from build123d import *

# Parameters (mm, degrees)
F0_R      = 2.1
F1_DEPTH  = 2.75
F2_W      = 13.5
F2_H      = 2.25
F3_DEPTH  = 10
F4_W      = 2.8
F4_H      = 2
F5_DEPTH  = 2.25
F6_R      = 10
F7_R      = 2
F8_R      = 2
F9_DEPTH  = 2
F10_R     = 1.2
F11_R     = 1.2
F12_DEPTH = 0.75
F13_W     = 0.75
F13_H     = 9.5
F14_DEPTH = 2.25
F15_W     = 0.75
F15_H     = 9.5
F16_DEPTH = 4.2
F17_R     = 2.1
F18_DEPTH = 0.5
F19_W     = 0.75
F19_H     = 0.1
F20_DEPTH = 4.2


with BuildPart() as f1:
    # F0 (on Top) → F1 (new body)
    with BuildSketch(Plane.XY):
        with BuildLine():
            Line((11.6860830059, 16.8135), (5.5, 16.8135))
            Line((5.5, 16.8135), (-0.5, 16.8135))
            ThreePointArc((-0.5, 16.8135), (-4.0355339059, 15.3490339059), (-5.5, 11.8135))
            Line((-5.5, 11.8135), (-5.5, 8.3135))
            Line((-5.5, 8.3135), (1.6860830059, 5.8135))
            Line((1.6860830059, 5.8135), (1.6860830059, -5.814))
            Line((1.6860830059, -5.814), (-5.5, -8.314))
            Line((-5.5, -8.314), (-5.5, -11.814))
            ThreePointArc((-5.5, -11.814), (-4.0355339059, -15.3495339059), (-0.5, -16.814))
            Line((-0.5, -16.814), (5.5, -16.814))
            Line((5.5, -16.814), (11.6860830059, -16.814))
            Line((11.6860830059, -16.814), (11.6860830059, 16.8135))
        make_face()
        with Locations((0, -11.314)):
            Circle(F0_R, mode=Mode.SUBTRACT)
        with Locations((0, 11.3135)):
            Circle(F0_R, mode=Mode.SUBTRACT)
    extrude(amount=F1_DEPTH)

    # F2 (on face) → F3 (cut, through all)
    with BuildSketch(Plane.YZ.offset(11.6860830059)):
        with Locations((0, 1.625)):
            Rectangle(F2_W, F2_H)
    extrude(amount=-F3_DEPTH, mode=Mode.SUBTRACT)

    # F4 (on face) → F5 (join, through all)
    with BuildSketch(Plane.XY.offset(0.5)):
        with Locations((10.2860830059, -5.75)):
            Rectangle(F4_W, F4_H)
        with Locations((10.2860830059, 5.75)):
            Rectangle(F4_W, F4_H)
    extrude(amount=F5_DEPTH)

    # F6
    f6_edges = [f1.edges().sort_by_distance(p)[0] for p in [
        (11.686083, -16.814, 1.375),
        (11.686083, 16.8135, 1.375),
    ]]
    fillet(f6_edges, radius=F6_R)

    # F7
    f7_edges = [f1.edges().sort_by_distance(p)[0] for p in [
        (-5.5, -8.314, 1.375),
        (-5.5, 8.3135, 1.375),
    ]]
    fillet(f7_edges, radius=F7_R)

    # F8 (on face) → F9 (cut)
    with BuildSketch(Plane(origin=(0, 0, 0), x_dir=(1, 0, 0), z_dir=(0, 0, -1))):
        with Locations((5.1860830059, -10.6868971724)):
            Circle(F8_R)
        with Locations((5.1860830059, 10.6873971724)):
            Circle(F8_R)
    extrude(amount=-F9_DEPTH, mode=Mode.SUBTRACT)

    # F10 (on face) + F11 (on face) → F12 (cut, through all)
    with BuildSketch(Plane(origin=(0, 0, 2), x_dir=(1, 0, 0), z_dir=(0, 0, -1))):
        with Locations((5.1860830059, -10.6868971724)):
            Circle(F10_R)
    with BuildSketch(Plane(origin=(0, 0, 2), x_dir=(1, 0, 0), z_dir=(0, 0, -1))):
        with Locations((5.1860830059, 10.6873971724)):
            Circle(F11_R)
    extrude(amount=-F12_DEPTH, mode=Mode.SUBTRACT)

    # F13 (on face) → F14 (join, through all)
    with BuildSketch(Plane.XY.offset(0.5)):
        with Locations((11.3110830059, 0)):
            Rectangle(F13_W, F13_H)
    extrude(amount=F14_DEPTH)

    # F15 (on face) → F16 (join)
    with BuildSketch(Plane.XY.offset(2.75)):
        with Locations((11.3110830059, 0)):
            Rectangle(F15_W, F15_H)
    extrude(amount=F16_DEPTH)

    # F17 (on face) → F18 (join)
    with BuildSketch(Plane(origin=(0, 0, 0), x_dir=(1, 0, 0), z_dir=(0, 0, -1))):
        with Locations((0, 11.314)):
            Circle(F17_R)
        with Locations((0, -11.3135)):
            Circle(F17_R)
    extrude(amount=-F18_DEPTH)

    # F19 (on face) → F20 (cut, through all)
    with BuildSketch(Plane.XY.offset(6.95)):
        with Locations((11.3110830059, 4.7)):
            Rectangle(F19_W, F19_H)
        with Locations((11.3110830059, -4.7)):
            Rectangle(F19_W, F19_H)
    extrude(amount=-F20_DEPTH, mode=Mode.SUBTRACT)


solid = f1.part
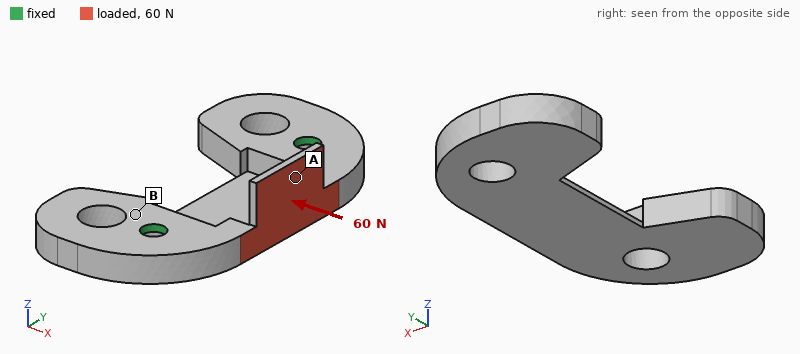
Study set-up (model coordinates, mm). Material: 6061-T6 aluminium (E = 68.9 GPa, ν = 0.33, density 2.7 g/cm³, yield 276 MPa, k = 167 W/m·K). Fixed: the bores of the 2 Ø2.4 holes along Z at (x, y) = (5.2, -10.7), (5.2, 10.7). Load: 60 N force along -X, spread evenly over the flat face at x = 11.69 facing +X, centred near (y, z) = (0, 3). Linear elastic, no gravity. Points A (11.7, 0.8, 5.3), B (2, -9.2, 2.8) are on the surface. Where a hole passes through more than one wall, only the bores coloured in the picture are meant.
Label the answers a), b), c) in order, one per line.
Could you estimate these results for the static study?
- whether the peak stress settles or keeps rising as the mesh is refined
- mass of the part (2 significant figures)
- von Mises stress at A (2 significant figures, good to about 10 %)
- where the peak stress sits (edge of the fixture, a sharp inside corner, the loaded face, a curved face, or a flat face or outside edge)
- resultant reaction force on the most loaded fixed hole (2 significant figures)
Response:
a) keeps rising
b) 2.2 g
c) 42 MPa
d) a sharp inside corner
e) 36 N
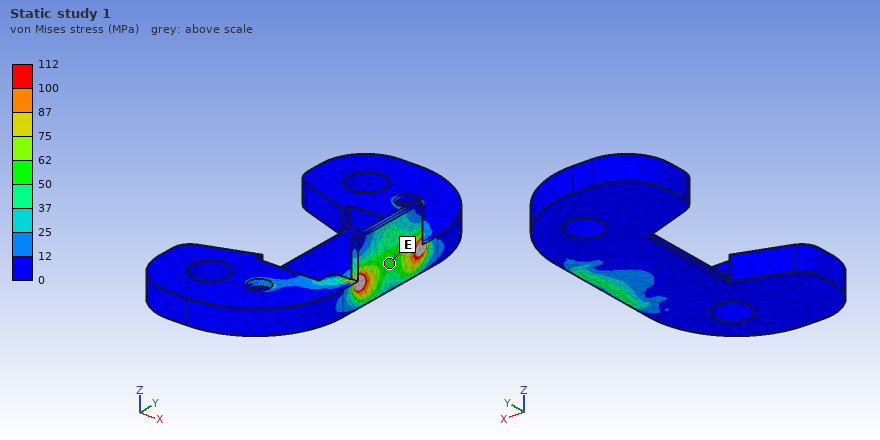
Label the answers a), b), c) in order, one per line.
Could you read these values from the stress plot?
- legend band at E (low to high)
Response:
a) 50 to 62 MPa
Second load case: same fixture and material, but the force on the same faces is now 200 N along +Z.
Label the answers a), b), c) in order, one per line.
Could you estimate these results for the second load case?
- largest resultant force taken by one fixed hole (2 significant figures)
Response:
a) 150 N
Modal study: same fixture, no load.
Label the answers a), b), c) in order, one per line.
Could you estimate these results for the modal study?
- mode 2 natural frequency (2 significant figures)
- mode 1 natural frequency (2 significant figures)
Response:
a) 11 kHz
b) 9200 Hz
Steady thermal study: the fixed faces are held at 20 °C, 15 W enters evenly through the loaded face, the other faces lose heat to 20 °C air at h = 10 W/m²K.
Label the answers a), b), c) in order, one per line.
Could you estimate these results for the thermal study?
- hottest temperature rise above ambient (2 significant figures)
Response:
a) 71 K
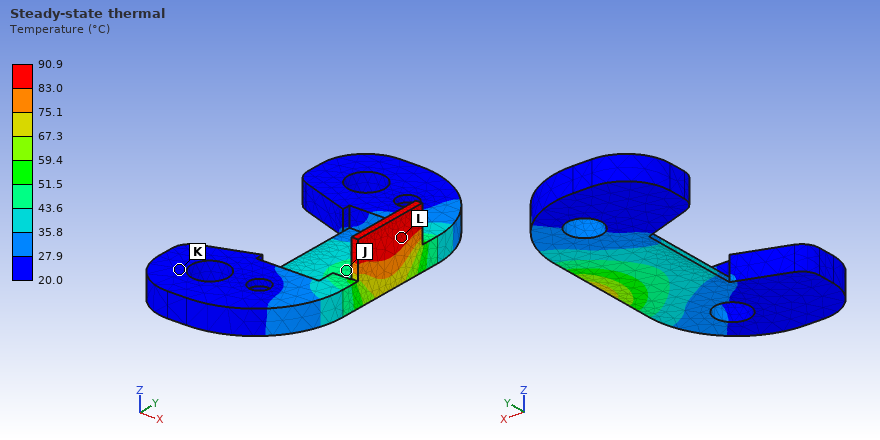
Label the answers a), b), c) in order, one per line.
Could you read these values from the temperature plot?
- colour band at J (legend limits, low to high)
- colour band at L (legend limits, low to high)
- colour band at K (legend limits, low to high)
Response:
a) 43.6 to 51.5 °C
b) 83.0 to 90.9 °C
c) 20.0 to 27.9 °C
